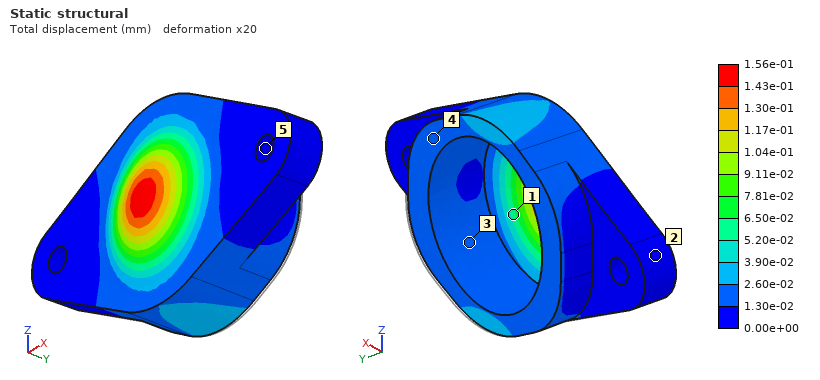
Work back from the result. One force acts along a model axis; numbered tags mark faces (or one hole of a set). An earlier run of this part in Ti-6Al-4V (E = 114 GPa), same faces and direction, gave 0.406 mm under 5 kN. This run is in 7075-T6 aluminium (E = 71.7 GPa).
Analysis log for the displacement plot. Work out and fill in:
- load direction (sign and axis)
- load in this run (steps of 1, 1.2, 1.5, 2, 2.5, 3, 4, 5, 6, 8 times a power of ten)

-Y
1.2 kN
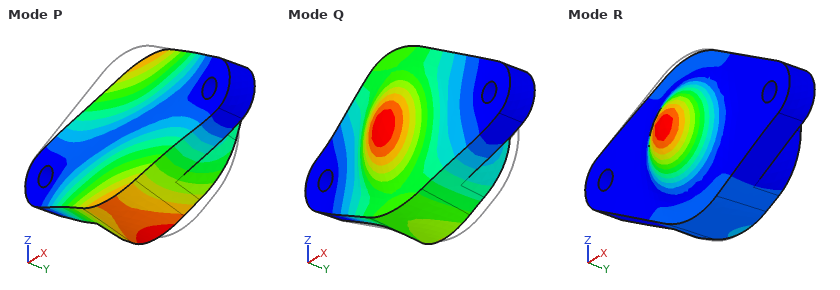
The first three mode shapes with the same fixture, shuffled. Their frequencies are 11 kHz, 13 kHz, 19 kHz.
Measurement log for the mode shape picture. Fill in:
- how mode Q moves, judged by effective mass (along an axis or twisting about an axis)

along Y
